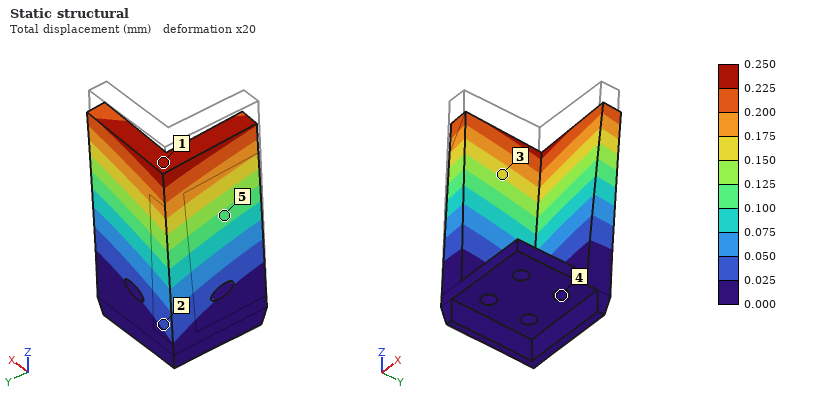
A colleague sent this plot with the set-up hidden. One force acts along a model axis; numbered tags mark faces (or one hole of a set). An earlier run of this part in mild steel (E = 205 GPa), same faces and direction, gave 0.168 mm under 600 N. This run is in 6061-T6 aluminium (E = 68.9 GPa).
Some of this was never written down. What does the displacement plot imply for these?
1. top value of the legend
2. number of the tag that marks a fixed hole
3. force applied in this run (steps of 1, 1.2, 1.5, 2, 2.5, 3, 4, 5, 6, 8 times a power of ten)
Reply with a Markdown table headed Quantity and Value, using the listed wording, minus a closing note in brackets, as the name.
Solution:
| Quantity | Value |
|---|---|
| top value of the legend | 0.250 mm |
| number of the tag that marks a fixed hole | 4 |
| force applied in this run | 300 N |
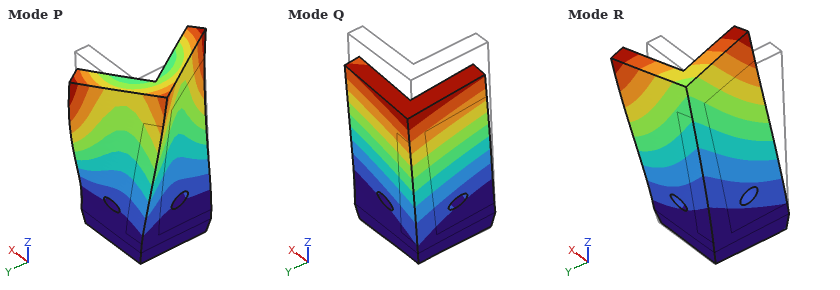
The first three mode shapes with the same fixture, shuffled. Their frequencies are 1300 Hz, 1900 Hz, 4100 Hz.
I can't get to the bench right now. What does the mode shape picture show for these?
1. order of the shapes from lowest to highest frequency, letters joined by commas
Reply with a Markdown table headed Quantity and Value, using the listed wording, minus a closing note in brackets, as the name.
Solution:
| Quantity | Value |
|---|---|
| order of the shapes from lowest to highest frequency, letters joined by commas | Q, R, P |
